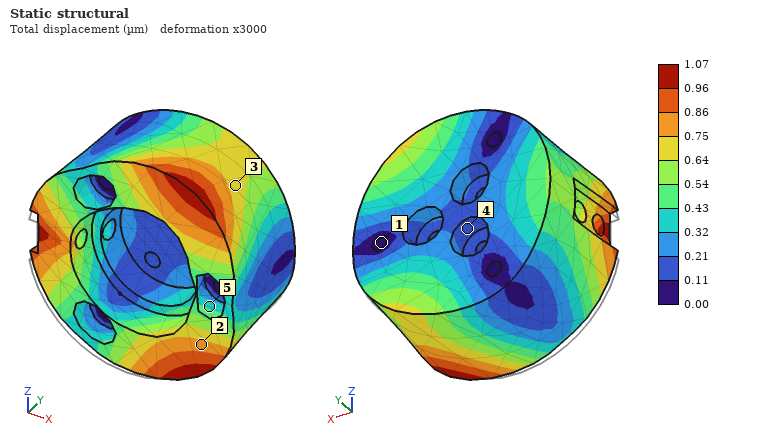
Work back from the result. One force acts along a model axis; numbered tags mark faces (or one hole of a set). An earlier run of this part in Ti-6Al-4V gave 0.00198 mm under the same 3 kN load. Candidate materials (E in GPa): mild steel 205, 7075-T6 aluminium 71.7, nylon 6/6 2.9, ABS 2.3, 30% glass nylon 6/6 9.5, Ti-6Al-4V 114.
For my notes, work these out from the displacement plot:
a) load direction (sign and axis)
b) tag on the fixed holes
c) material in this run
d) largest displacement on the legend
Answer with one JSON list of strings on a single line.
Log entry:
["+Y", "1", "mild steel", "1.07 µm"]
